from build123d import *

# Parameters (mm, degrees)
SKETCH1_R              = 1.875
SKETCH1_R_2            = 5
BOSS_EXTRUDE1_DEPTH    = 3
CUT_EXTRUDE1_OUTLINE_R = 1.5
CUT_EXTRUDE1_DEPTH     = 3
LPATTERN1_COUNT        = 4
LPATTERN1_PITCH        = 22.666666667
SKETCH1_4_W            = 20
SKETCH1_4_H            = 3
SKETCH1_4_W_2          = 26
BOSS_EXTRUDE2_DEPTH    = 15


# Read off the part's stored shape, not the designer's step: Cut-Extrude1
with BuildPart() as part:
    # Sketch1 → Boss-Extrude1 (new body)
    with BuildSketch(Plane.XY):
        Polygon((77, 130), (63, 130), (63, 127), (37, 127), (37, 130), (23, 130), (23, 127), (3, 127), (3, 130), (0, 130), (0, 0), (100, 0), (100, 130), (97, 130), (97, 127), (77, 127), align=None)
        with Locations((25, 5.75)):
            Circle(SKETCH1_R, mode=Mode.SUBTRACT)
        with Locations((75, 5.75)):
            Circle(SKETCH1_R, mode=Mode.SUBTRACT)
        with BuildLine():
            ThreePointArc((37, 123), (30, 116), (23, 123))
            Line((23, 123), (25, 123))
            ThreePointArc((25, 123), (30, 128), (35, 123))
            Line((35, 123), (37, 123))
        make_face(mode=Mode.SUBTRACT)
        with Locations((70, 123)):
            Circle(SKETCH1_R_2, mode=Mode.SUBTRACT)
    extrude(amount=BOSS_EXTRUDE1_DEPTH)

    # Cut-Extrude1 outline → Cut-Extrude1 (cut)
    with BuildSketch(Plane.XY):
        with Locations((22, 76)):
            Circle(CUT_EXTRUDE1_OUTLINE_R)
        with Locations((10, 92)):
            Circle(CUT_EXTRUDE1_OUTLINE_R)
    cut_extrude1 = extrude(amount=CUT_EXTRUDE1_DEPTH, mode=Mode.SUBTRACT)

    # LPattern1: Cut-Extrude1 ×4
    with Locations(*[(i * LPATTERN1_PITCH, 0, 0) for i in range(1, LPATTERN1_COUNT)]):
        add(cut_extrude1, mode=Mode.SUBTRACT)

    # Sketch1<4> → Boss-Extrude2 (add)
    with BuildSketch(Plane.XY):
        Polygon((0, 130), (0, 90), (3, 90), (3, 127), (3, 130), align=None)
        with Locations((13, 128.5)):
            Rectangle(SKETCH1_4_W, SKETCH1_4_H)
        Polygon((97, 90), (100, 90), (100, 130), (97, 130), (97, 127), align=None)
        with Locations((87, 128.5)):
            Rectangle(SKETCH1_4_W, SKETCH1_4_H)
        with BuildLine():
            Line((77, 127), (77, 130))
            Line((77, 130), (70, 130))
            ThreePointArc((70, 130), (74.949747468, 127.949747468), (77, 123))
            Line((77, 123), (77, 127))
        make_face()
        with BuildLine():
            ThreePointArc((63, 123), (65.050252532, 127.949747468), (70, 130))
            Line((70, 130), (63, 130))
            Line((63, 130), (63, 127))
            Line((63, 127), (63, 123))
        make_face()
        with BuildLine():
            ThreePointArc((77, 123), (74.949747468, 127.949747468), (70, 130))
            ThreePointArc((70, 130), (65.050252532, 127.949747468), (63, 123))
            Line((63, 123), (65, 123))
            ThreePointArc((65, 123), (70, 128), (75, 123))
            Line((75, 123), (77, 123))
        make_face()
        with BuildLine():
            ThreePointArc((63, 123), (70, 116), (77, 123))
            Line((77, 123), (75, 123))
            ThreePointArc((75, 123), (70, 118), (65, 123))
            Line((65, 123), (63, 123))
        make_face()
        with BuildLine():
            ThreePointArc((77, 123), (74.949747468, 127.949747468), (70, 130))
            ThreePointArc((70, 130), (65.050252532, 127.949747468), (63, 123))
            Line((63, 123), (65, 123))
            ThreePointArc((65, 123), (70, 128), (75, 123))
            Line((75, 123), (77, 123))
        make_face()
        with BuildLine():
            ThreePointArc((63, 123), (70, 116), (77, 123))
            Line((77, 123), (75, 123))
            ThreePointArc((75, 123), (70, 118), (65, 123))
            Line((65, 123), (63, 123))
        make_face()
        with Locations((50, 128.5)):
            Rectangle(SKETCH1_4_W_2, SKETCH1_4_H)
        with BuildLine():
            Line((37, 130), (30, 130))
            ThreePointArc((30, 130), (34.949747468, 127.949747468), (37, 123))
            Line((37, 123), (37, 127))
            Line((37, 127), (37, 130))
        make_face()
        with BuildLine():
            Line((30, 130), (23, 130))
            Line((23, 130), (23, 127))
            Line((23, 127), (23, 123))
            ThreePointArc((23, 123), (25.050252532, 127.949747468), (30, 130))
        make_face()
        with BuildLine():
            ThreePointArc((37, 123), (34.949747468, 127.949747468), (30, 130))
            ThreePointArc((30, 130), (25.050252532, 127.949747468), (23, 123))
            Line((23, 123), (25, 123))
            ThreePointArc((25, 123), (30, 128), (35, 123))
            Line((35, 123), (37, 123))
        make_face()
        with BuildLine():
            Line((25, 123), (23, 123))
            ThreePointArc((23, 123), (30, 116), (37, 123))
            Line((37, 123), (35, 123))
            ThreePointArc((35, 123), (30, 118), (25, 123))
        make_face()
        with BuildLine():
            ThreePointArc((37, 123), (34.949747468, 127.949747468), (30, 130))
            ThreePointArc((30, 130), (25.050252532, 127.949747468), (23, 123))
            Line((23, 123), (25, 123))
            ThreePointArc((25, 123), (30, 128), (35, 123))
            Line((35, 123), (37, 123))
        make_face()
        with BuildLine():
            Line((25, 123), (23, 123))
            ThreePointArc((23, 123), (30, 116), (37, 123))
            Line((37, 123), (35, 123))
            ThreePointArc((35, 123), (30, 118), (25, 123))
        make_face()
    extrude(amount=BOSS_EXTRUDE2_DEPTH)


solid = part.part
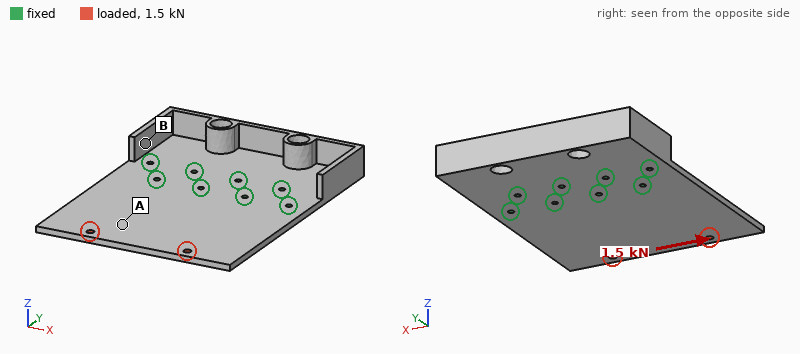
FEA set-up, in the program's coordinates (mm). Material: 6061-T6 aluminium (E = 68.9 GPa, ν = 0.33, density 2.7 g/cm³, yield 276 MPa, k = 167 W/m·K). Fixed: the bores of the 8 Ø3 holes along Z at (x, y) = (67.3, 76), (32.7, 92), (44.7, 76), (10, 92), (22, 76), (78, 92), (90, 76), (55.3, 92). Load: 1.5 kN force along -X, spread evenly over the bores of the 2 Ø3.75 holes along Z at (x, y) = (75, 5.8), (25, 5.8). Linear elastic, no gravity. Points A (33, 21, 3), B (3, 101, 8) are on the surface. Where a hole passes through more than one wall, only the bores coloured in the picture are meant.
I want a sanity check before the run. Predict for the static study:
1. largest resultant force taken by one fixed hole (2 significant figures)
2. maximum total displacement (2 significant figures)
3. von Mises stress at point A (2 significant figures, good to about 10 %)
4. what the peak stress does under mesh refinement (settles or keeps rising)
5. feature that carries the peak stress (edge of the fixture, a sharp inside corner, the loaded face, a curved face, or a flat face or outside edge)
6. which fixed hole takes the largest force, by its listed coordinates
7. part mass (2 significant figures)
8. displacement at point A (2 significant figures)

1.1 kN
37 µm
11 MPa
keeps rising
edge of the fixture
(90, 76)
120 g
23 µm
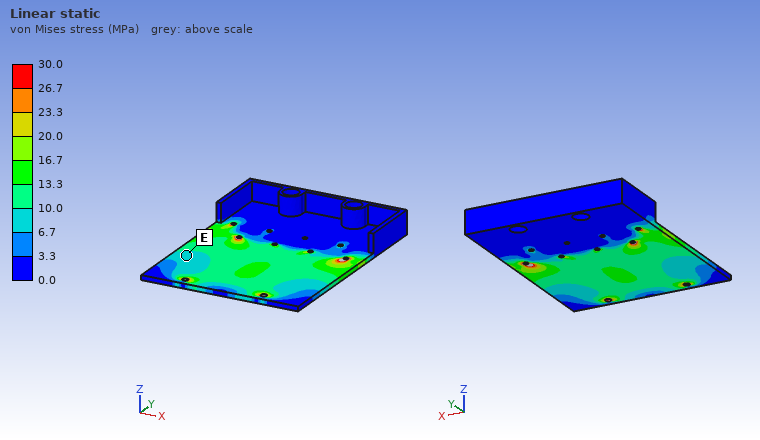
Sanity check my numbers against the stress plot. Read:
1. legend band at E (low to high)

6.7 to 10.0 MPa
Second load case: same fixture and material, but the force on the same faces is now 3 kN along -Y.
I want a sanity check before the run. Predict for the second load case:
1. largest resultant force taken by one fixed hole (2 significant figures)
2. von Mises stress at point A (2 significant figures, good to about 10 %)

610 N
16 MPa
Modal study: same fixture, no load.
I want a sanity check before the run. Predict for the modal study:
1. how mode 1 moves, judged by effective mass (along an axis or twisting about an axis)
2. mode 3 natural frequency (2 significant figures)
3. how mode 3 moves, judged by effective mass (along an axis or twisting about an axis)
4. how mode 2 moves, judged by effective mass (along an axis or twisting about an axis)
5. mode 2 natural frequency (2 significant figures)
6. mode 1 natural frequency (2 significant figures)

along Z
1200 Hz
along Z
twisting about Y
830 Hz
430 Hz
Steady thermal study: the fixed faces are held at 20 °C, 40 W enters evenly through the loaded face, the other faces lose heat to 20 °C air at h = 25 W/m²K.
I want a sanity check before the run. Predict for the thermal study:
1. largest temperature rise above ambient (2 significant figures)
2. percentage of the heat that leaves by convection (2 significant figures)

61 K
26 %
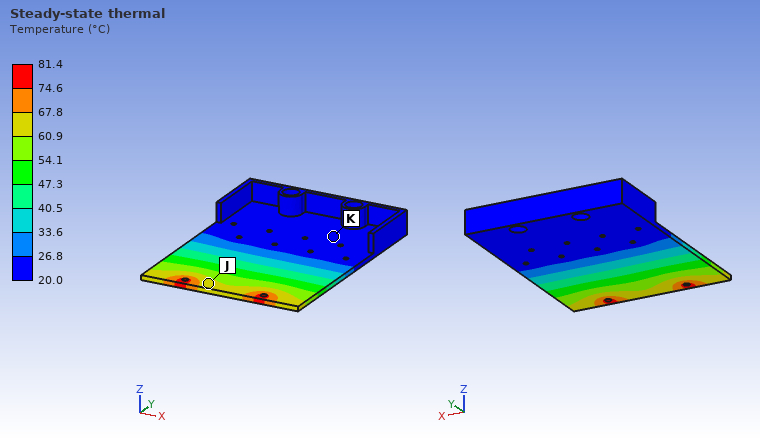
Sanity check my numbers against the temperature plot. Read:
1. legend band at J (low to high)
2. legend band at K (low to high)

60.9 to 67.8 °C
20.0 to 26.8 °C
